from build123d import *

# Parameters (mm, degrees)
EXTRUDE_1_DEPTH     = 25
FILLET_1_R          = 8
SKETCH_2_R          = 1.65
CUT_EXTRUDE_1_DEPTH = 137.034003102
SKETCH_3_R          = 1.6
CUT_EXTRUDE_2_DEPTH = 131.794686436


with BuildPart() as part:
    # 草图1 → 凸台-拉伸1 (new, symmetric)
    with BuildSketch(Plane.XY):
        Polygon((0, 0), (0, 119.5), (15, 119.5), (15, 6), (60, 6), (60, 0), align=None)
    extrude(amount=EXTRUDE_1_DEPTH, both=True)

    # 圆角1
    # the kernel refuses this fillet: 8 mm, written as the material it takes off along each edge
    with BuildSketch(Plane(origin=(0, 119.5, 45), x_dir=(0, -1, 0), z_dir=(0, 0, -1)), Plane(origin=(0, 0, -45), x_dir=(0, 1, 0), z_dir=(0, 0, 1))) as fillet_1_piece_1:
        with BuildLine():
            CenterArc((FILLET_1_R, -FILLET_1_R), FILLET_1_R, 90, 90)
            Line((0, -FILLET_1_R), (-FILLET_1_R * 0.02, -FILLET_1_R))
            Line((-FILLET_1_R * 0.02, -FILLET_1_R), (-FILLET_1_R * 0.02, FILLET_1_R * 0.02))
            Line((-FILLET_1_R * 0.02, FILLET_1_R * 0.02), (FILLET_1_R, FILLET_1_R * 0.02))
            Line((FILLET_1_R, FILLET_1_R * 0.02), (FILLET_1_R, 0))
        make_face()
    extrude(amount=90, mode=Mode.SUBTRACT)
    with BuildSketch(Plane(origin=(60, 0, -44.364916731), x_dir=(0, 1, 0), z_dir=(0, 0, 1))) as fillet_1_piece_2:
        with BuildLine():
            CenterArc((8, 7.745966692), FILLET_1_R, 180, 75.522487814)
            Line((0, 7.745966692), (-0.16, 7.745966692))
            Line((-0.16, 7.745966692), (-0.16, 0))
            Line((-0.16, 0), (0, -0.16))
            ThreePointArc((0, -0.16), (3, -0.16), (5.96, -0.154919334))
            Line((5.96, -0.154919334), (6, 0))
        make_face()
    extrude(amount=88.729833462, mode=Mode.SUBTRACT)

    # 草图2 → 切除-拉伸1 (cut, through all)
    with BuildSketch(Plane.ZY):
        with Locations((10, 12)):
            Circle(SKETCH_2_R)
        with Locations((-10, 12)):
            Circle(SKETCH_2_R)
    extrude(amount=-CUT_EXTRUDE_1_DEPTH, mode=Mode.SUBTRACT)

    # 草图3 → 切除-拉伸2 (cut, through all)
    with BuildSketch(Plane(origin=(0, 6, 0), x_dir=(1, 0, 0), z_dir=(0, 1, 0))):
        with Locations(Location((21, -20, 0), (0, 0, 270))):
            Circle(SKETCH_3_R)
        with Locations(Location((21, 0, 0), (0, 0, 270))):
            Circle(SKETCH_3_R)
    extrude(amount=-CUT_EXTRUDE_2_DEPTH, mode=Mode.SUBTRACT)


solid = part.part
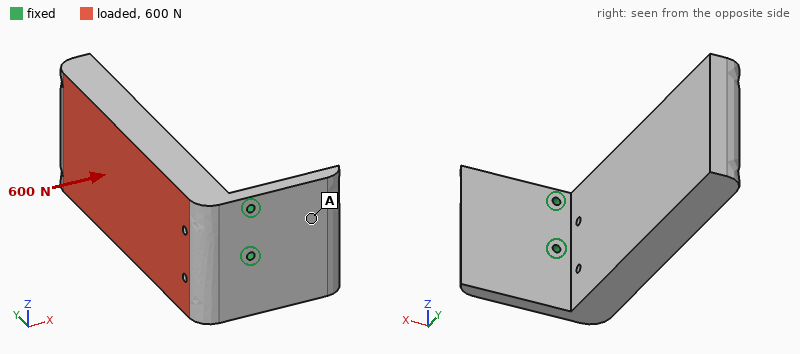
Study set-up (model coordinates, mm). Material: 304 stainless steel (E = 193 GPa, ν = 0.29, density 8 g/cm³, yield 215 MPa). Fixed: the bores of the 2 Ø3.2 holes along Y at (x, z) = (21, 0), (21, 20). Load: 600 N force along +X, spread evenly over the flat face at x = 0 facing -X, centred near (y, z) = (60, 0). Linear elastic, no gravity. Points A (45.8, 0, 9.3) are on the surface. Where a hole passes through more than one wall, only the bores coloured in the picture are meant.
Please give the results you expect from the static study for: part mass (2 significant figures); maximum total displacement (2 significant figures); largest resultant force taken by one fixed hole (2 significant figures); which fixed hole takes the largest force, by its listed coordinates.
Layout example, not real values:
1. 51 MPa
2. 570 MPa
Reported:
1. 810 g
2. 0.33 mm
3. 580 N
4. (21, 0)
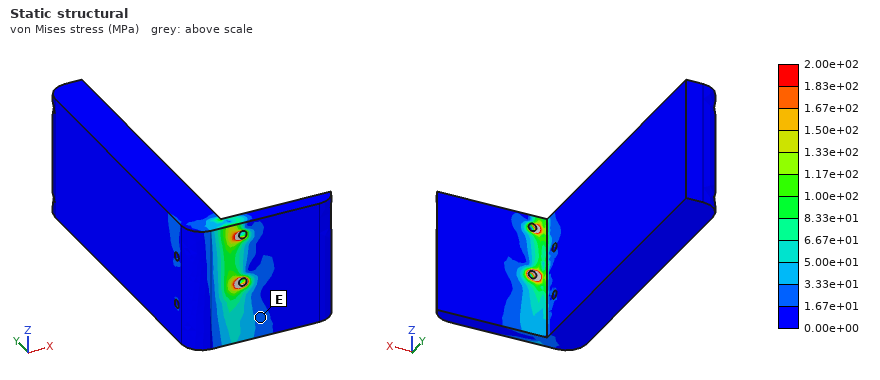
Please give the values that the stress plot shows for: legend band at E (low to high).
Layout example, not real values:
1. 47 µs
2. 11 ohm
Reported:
1. 1.67e+01 to 3.33e+01 MPa
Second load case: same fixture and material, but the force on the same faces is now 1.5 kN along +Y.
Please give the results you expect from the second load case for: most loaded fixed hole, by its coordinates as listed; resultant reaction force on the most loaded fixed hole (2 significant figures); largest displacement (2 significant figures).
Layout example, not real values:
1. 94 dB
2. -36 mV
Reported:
1. (21, 0)
2. 1.4 kN
3. 0.25 mm
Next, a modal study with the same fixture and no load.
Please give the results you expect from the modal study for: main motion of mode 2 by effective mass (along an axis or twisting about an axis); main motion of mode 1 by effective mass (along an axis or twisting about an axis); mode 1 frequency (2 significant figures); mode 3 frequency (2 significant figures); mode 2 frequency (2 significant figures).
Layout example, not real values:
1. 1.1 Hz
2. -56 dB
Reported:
1. along Z
2. along X
3. 310 Hz
4. 2900 Hz
5. 760 Hz
